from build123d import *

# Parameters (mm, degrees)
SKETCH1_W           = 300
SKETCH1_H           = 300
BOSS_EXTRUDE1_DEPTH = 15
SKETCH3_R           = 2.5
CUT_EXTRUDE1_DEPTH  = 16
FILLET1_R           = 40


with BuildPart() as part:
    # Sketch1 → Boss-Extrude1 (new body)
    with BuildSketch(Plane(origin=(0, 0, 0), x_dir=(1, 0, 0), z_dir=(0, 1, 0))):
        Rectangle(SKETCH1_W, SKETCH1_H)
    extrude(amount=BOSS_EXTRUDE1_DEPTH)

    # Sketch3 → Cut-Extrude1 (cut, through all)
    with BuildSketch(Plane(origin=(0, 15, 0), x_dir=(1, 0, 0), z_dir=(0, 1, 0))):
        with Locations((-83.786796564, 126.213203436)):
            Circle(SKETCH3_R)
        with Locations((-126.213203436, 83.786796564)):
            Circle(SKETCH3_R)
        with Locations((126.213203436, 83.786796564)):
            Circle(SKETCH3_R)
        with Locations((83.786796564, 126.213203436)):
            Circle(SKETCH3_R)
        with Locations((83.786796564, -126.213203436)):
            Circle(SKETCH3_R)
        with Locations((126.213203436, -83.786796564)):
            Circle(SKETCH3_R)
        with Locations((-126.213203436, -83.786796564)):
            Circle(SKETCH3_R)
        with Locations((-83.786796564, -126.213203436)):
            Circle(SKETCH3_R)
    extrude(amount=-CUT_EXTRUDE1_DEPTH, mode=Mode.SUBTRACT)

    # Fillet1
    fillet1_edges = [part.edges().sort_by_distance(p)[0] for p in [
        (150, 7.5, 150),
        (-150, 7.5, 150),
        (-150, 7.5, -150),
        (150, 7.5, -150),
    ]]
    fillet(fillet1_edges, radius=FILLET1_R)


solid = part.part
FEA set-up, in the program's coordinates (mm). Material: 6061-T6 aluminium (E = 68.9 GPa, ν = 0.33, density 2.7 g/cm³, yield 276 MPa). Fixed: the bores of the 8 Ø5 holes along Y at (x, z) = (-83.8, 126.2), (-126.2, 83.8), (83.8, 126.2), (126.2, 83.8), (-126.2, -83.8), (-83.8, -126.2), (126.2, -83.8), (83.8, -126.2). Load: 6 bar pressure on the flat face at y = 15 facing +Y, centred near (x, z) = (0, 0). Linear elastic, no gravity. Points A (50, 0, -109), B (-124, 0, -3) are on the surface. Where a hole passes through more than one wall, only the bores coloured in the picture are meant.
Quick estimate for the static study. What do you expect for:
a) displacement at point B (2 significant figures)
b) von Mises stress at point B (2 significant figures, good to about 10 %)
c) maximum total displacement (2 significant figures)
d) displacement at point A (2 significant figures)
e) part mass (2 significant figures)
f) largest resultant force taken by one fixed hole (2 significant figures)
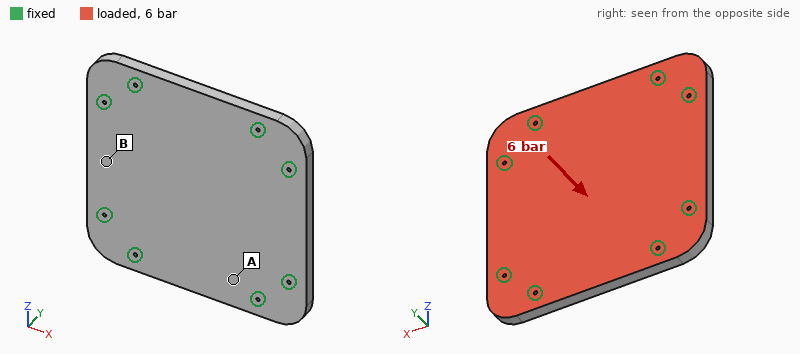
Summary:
0.16 mm
33 MPa
0.42 mm
0.12 mm
3.6 kg
6.6 kN
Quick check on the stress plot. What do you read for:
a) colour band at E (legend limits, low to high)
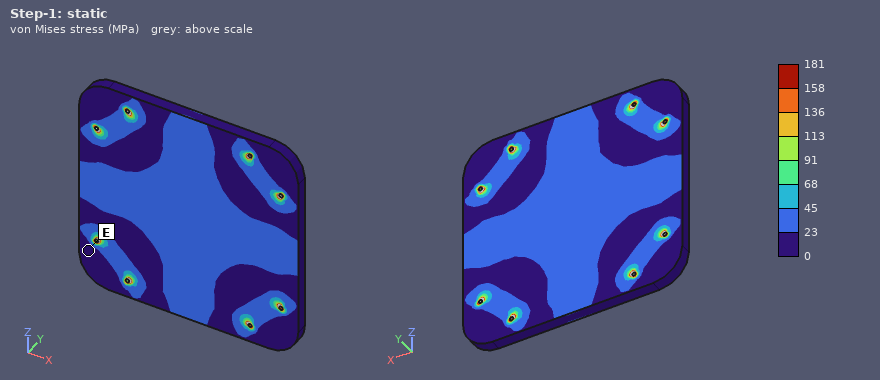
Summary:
0 to 23 MPa
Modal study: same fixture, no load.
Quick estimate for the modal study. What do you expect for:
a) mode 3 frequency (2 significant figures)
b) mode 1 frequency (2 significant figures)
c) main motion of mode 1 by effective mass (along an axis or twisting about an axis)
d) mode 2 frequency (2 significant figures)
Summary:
2200 Hz
1200 Hz
along Y
2200 Hz
